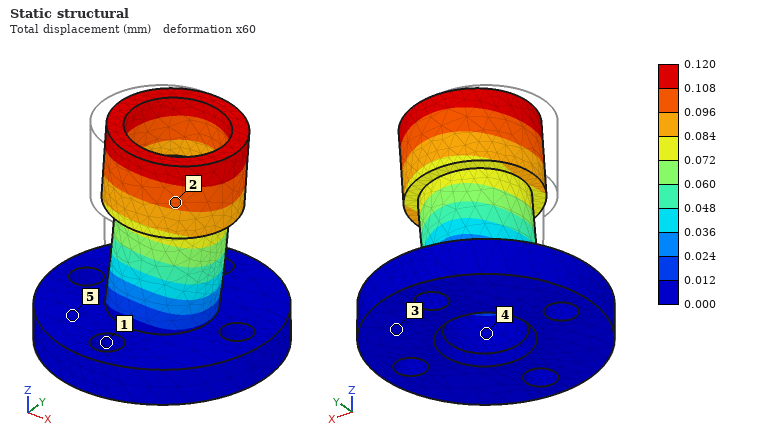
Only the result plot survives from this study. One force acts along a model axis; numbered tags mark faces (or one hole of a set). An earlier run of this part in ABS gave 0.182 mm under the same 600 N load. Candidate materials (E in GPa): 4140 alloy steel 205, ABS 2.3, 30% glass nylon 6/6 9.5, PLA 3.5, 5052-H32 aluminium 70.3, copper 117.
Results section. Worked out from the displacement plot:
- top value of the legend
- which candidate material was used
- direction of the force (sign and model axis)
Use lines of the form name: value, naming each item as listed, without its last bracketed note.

top value of the legend: 0.120 mm
which candidate material was used: PLA
direction of the force: +X
